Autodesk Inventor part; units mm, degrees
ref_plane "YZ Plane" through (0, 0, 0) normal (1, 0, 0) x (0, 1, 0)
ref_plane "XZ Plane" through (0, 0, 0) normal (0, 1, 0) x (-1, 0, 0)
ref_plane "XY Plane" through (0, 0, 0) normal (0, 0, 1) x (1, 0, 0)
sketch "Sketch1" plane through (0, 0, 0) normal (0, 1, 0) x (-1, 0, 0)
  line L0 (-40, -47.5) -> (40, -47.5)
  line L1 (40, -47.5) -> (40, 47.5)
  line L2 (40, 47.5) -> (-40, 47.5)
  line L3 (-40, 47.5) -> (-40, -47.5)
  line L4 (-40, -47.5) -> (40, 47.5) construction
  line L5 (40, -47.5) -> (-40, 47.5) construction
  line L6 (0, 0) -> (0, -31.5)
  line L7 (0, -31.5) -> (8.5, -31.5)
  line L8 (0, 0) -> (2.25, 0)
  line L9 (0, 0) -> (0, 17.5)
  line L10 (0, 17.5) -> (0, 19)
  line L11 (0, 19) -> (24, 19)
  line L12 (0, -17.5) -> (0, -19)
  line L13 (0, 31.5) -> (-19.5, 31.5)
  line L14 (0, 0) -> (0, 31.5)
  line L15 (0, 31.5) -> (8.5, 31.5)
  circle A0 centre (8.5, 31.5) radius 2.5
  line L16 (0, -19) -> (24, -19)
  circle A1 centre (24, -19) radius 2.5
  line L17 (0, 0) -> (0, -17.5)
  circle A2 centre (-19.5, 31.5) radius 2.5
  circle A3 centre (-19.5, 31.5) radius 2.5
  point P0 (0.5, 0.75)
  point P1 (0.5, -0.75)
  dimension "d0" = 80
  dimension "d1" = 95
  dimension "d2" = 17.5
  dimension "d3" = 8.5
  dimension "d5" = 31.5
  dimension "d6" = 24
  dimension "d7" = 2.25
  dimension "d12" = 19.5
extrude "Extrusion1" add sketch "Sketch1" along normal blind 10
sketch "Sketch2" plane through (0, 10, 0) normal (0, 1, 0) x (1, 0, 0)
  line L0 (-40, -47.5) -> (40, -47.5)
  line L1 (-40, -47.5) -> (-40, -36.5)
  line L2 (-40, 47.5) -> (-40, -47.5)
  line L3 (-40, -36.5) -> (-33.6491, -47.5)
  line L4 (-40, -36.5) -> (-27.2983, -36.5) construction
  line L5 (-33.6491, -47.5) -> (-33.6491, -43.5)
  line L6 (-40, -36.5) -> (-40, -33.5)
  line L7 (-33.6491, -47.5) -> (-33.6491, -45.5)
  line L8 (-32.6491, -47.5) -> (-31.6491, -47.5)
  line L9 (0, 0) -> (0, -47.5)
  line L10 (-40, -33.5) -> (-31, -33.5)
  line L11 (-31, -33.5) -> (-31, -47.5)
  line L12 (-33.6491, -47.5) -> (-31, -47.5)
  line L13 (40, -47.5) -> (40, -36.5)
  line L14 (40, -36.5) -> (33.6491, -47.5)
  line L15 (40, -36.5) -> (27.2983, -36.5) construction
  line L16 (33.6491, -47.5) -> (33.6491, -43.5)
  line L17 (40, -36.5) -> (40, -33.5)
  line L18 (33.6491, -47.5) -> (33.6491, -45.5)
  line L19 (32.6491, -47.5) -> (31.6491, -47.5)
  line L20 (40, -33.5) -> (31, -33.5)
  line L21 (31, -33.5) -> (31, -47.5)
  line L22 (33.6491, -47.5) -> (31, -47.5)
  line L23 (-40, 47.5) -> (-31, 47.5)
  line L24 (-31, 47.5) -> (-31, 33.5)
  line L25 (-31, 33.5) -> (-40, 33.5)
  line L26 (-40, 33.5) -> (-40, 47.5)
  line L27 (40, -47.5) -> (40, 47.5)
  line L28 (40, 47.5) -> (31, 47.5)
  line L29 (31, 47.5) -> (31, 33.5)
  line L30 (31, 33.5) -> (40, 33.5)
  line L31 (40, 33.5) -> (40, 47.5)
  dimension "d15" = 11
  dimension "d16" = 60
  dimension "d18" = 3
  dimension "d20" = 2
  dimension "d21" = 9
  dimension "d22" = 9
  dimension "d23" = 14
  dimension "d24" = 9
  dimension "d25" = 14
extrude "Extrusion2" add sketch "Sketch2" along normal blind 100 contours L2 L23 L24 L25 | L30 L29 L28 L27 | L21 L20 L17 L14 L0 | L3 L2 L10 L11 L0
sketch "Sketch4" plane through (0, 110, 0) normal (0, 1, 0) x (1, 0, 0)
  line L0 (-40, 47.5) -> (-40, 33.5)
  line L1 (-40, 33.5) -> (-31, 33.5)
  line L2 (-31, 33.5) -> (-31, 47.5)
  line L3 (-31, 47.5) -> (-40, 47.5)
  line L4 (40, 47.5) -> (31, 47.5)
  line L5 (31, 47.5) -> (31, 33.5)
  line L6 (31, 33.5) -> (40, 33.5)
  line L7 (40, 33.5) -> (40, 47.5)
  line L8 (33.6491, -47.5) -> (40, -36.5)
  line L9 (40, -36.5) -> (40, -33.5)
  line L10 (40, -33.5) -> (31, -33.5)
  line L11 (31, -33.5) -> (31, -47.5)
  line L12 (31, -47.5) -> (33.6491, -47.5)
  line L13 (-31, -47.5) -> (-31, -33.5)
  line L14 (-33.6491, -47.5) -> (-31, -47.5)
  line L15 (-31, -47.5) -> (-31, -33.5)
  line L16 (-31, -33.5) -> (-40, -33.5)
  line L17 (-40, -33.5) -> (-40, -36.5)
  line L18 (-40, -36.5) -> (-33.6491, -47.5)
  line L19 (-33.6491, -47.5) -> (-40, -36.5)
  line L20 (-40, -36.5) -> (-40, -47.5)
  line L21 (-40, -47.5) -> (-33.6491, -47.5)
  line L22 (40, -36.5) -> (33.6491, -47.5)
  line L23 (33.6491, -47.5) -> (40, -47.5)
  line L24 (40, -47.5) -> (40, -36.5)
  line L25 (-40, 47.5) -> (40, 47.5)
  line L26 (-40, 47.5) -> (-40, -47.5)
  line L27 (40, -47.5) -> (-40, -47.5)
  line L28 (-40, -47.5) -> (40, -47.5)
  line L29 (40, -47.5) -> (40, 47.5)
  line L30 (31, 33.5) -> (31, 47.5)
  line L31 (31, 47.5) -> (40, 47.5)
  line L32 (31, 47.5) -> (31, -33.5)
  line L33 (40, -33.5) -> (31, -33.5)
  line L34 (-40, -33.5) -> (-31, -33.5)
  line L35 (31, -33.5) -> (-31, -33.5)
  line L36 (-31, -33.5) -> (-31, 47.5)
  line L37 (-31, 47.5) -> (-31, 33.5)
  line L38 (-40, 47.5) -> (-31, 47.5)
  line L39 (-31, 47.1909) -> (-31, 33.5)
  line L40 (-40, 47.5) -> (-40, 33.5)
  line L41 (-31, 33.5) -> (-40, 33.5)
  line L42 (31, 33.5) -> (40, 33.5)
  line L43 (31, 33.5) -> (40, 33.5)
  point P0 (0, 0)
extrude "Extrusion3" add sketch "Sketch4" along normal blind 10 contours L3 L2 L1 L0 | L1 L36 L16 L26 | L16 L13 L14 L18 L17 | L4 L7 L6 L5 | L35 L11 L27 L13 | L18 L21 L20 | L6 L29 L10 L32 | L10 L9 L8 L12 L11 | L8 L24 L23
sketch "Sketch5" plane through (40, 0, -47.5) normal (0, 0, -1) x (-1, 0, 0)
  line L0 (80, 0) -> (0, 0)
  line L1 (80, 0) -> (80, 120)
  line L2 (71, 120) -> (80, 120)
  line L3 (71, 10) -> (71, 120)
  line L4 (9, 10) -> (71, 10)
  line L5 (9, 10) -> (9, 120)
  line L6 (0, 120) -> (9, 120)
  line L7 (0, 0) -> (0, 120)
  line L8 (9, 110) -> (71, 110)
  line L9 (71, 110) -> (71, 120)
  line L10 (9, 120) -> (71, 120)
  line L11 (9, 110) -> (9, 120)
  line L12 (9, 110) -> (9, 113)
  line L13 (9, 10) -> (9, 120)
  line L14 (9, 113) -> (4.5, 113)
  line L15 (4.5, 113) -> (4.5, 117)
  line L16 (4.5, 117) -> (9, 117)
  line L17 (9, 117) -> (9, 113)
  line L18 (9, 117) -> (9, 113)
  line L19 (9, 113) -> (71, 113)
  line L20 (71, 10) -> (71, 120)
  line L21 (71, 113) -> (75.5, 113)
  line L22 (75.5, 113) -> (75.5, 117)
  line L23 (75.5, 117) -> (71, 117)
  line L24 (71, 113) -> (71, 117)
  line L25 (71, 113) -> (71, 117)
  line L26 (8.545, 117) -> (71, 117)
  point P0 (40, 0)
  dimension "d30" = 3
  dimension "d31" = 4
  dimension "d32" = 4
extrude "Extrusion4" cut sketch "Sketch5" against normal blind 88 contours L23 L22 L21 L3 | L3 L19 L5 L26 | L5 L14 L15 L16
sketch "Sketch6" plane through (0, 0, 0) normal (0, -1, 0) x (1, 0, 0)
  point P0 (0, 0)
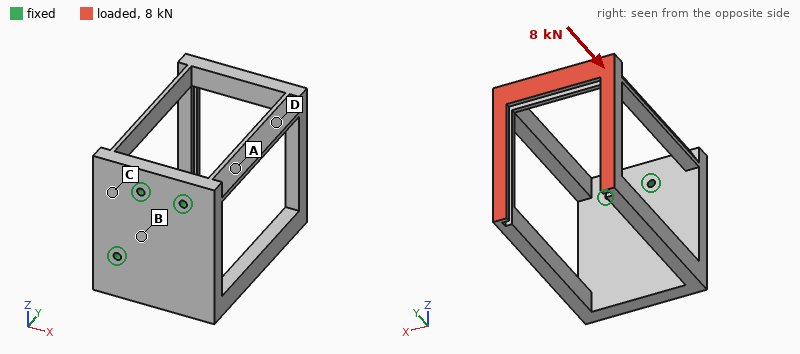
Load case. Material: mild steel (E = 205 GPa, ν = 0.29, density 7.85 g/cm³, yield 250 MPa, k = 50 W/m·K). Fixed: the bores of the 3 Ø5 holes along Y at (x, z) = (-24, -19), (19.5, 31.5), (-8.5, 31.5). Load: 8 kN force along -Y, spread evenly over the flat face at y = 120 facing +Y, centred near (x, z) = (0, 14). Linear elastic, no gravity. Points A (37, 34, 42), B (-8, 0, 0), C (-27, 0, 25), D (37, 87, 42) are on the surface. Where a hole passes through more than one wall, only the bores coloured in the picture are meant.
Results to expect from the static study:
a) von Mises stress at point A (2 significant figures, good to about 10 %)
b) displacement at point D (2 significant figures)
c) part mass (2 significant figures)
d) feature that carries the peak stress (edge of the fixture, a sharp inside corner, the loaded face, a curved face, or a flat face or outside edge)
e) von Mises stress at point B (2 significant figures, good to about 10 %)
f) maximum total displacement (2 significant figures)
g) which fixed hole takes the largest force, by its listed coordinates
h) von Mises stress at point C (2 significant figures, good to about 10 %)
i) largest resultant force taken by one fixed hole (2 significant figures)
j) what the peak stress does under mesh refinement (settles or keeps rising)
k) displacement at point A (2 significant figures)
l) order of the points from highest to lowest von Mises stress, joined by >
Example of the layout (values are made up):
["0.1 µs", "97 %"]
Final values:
["23 MPa", "0.053 mm", "1.1 kg", "edge of the fixture", "34 MPa", "0.12 mm", "(19.5, 31.5)", "48 MPa", "3.4 kN", "keeps rising", "0.035 mm", "C > B > A > D"]
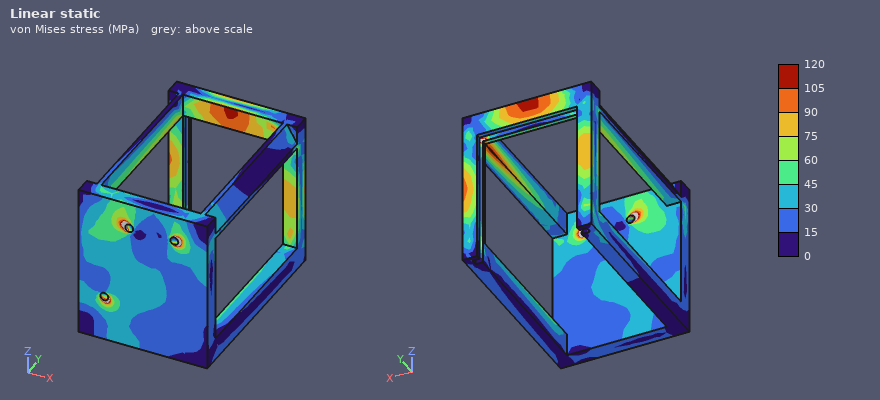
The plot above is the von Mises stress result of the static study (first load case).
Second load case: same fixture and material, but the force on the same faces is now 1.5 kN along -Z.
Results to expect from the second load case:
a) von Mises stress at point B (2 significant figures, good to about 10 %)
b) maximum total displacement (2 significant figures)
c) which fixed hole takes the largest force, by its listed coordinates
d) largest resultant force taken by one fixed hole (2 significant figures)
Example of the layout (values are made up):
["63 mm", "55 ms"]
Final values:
["18 MPa", "0.35 mm", "(-24, -19)", "2.0 kN"]
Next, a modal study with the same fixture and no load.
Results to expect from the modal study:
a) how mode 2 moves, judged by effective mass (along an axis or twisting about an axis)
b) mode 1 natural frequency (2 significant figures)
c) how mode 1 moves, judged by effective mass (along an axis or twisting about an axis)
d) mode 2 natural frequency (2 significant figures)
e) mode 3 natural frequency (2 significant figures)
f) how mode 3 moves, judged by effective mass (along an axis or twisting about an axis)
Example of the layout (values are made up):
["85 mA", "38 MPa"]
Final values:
["along Z", "450 Hz", "along X", "660 Hz", "830 Hz", "twisting about Y"]
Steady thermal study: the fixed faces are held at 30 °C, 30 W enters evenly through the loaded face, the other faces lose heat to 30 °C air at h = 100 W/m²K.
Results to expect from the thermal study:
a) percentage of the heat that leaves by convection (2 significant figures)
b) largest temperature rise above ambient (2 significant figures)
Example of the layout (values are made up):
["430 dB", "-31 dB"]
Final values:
["98 %", "28 K"]
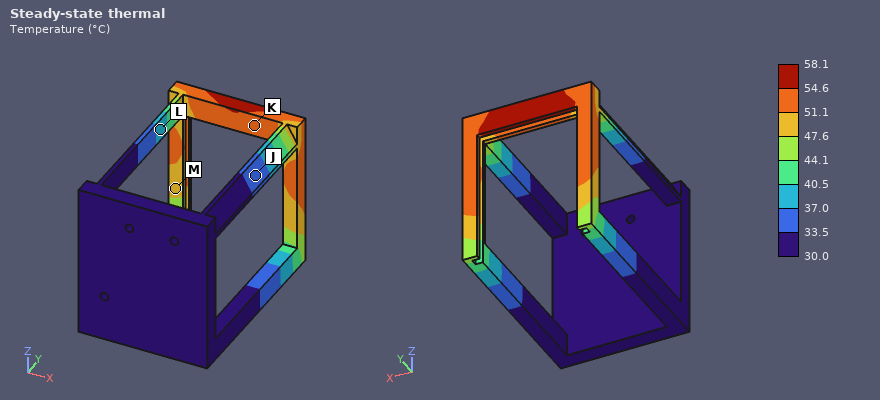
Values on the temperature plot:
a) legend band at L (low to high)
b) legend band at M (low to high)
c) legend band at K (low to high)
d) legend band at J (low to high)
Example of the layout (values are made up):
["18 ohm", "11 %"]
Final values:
["37.0 to 40.5 °C", "47.6 to 51.1 °C", "51.1 to 54.6 °C", "33.5 to 37.0 °C"]
